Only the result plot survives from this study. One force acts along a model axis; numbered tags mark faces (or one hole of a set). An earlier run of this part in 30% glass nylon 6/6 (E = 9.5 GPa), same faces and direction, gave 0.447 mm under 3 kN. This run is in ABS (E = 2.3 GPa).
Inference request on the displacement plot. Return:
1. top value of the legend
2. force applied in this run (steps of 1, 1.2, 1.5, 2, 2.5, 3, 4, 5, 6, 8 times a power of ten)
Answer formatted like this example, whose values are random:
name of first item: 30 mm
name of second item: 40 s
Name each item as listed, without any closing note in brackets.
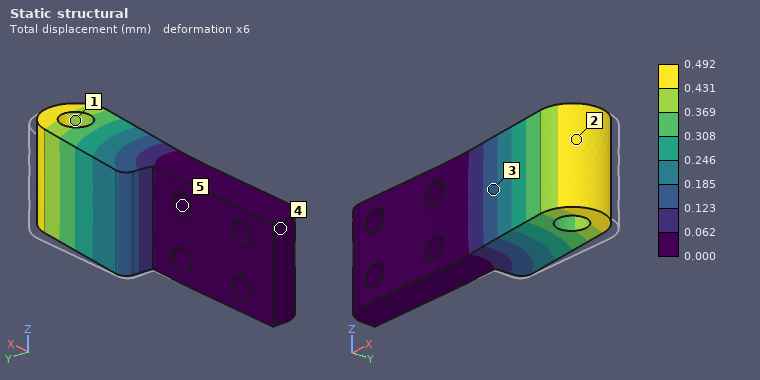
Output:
top value of the legend: 0.492 mm
force applied in this run: 800 N
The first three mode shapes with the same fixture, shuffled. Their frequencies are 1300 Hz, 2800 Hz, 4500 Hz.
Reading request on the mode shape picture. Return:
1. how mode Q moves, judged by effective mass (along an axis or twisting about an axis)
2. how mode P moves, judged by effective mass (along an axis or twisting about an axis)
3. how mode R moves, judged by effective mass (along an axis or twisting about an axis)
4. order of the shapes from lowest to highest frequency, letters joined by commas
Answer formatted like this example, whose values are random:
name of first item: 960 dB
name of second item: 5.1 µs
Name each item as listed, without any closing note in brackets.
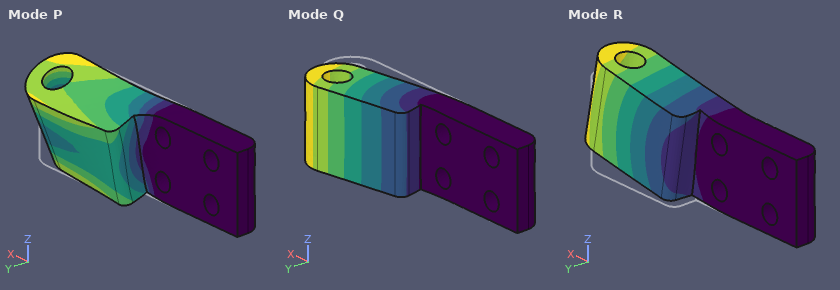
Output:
how mode Q moves, judged by effective mass: along Y
how mode P moves, judged by effective mass: twisting about X
how mode R moves, judged by effective mass: along Z
order of the shapes from lowest to highest frequency, letters joined by commas: Q, R, P
